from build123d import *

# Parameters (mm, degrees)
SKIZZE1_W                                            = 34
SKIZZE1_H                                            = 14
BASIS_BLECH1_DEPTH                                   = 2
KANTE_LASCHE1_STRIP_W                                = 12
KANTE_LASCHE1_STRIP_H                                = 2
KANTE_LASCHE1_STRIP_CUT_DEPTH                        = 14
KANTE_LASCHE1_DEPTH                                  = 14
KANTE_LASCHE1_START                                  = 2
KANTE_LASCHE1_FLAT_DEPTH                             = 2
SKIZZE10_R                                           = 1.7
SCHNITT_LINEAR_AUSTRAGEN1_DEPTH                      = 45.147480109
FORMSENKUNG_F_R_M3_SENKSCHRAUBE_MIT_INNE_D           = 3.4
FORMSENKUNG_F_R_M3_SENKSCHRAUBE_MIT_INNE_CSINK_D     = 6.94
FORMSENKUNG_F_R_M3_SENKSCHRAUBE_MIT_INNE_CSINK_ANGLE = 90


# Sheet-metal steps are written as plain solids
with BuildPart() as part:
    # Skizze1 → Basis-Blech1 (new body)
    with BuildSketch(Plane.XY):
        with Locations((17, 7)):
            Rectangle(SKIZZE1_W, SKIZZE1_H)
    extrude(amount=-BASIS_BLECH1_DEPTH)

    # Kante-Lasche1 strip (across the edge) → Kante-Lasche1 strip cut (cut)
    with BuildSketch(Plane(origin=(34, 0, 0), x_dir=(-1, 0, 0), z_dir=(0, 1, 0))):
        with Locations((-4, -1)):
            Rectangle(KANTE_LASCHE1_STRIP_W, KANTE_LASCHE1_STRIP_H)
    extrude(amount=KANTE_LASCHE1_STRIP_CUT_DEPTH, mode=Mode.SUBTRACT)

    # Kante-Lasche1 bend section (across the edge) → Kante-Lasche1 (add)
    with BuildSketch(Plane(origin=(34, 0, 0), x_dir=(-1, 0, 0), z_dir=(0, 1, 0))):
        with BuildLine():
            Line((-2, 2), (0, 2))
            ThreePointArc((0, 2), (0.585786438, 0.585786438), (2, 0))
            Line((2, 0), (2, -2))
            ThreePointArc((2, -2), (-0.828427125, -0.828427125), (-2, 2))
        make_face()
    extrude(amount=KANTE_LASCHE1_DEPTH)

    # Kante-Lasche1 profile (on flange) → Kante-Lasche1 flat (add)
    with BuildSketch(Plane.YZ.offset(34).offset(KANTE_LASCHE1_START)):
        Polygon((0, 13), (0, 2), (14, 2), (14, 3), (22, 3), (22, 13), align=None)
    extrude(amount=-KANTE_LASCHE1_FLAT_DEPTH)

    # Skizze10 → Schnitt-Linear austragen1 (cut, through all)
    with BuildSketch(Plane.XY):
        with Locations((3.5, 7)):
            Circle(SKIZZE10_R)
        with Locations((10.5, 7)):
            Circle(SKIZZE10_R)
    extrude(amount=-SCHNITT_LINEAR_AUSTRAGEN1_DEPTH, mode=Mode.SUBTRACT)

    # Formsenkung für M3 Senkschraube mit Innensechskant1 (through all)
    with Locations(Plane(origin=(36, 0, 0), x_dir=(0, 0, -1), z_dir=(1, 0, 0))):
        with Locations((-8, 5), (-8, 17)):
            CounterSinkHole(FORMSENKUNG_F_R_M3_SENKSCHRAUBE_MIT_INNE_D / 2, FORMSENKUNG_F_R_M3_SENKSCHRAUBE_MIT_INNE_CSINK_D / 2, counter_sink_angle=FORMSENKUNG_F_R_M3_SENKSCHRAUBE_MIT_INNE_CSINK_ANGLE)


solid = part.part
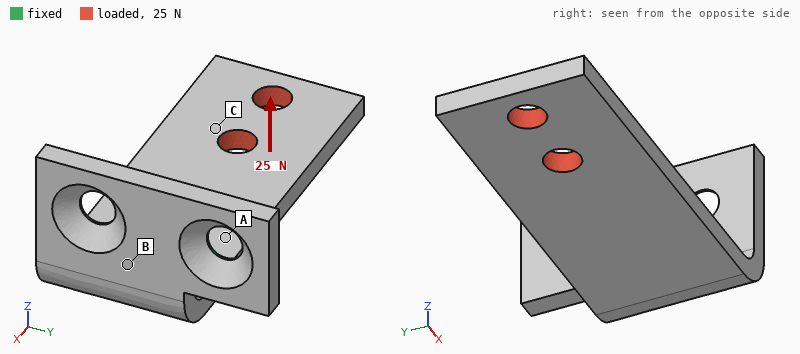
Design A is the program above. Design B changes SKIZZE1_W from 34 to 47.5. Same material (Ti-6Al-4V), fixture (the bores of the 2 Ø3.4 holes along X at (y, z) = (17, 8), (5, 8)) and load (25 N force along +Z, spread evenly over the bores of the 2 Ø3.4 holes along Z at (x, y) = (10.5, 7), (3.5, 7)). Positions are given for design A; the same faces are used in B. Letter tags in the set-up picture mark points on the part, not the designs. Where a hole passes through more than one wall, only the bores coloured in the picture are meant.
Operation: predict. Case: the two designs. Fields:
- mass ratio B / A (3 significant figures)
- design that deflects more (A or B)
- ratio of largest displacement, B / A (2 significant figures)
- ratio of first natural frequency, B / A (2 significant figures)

1.14
B
1.2
0.73
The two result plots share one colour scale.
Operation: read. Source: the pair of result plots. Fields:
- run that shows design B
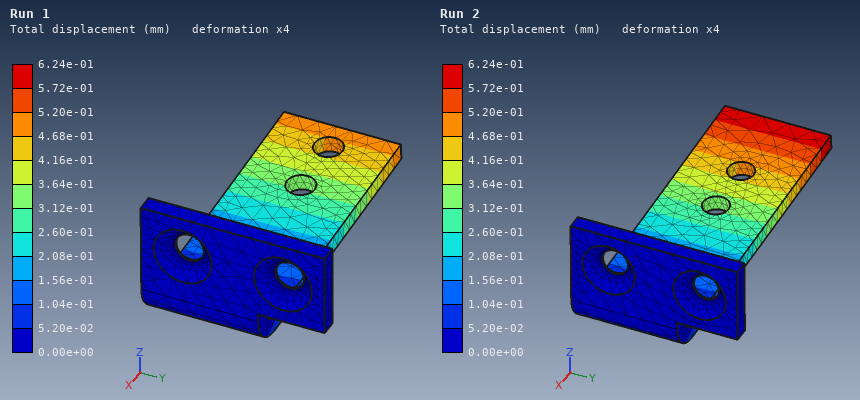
Run 2
